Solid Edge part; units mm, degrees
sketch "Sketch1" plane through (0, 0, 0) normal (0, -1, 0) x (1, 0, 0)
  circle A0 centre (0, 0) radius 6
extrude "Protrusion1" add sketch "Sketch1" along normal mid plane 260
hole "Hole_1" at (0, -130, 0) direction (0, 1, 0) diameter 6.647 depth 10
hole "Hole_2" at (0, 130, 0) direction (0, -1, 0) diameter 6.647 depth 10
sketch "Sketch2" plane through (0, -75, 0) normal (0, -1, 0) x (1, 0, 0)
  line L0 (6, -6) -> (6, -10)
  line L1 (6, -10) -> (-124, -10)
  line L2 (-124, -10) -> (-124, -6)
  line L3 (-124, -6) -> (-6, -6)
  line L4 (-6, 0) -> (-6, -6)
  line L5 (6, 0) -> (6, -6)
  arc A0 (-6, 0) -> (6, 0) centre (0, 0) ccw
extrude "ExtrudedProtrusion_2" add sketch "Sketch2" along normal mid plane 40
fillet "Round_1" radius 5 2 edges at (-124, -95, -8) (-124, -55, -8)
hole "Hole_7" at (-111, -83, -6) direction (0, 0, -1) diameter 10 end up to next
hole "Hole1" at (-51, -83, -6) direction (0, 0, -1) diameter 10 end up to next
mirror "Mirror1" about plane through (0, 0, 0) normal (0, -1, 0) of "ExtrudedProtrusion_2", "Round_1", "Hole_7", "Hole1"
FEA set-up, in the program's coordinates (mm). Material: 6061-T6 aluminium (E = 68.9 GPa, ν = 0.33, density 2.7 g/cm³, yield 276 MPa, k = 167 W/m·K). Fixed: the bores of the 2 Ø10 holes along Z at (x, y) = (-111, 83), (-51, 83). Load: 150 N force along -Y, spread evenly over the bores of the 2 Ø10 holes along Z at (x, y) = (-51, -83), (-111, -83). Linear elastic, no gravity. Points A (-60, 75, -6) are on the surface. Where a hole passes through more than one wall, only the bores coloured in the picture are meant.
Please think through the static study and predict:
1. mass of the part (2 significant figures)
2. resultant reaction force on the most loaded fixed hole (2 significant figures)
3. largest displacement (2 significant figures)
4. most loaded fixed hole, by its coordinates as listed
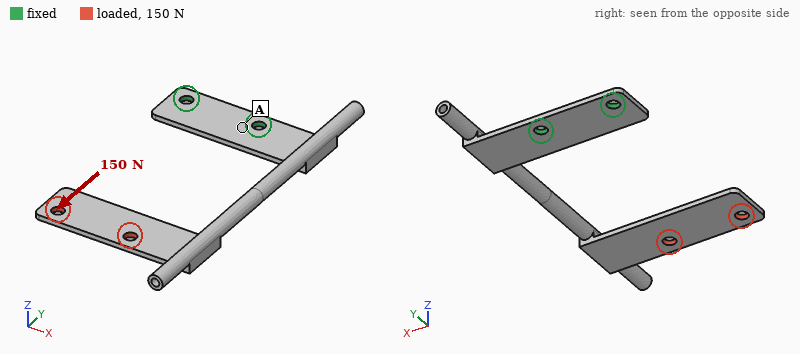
190 g
120 N
3.5 mm
(-51, 83)
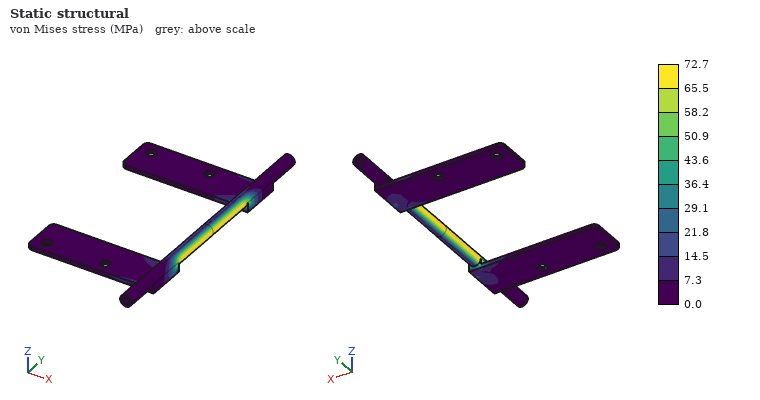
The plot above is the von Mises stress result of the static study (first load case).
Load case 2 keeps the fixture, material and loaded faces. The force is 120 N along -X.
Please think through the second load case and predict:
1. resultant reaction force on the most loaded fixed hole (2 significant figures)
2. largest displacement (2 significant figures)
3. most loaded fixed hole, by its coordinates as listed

360 N
3.2 mm
(-111, 83)
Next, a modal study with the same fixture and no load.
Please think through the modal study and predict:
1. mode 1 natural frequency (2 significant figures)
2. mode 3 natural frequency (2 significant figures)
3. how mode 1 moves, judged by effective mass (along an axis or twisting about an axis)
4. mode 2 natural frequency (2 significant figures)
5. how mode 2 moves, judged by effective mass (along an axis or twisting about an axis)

69 Hz
150 Hz
along Z
120 Hz
along X
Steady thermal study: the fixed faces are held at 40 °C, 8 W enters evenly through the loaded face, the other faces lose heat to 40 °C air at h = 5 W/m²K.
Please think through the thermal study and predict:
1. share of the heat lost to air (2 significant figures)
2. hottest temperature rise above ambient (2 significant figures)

49 %
58 K
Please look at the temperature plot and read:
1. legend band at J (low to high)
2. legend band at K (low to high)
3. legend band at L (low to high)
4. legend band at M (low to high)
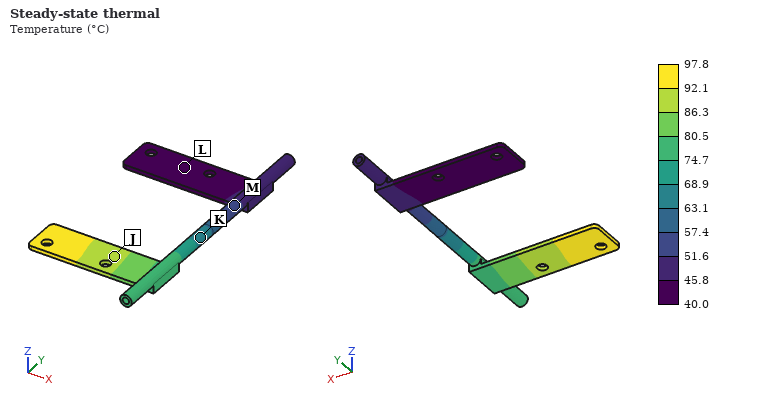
86.3 to 92.1 °C
63.1 to 68.9 °C
40.0 to 45.8 °C
51.6 to 57.4 °C
